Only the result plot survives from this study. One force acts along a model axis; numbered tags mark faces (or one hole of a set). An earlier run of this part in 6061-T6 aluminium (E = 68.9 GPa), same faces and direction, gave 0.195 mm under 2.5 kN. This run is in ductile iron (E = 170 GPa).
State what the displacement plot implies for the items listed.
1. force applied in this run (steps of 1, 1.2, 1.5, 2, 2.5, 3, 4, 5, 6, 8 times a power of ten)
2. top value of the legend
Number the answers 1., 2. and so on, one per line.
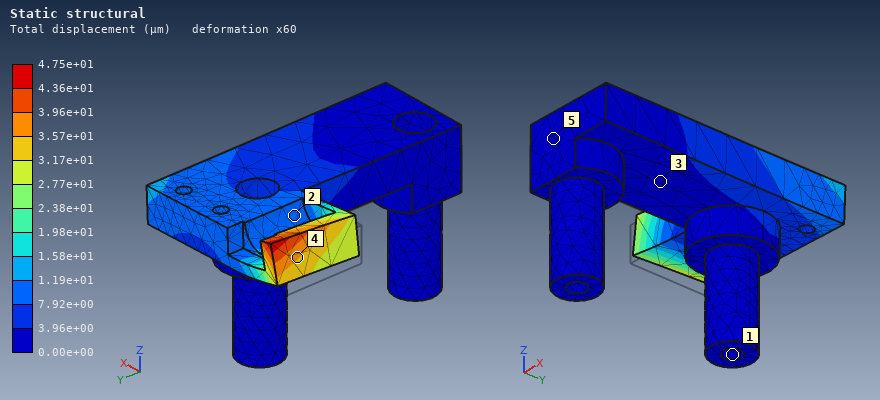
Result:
1. 1.5 kN
2. 4.75e+01 µm
